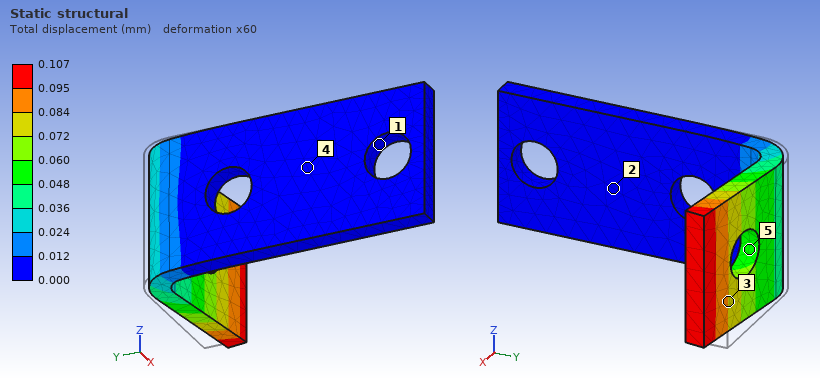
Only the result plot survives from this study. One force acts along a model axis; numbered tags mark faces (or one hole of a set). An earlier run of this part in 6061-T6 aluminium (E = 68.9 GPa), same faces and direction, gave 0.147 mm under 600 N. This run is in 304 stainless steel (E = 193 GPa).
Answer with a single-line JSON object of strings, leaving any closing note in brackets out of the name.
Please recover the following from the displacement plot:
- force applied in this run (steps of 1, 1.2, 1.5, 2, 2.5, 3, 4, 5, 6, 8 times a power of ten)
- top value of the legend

{"force applied in this run": "1.2 kN", "top value of the legend": "0.107 mm"}
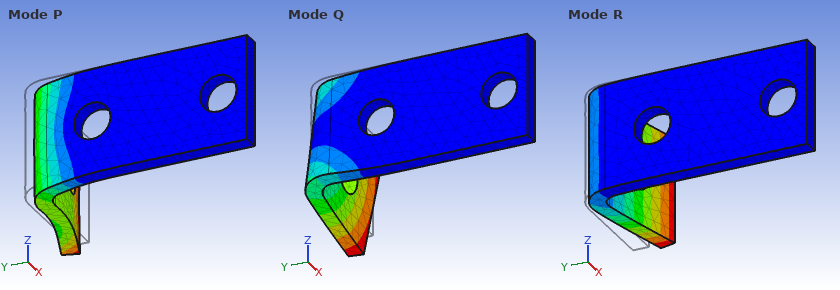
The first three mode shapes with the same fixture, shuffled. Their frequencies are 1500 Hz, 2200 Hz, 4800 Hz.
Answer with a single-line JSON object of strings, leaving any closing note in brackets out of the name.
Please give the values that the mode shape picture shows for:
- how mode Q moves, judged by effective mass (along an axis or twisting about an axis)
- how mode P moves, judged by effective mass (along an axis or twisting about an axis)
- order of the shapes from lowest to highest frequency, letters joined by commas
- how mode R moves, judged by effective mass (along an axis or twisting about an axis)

{"how mode Q moves, judged by effective mass": "along Z", "how mode P moves, judged by effective mass": "along X", "order of the shapes from lowest to highest frequency, letters joined by commas": "R, Q, P", "how mode R moves, judged by effective mass": "along Y"}
